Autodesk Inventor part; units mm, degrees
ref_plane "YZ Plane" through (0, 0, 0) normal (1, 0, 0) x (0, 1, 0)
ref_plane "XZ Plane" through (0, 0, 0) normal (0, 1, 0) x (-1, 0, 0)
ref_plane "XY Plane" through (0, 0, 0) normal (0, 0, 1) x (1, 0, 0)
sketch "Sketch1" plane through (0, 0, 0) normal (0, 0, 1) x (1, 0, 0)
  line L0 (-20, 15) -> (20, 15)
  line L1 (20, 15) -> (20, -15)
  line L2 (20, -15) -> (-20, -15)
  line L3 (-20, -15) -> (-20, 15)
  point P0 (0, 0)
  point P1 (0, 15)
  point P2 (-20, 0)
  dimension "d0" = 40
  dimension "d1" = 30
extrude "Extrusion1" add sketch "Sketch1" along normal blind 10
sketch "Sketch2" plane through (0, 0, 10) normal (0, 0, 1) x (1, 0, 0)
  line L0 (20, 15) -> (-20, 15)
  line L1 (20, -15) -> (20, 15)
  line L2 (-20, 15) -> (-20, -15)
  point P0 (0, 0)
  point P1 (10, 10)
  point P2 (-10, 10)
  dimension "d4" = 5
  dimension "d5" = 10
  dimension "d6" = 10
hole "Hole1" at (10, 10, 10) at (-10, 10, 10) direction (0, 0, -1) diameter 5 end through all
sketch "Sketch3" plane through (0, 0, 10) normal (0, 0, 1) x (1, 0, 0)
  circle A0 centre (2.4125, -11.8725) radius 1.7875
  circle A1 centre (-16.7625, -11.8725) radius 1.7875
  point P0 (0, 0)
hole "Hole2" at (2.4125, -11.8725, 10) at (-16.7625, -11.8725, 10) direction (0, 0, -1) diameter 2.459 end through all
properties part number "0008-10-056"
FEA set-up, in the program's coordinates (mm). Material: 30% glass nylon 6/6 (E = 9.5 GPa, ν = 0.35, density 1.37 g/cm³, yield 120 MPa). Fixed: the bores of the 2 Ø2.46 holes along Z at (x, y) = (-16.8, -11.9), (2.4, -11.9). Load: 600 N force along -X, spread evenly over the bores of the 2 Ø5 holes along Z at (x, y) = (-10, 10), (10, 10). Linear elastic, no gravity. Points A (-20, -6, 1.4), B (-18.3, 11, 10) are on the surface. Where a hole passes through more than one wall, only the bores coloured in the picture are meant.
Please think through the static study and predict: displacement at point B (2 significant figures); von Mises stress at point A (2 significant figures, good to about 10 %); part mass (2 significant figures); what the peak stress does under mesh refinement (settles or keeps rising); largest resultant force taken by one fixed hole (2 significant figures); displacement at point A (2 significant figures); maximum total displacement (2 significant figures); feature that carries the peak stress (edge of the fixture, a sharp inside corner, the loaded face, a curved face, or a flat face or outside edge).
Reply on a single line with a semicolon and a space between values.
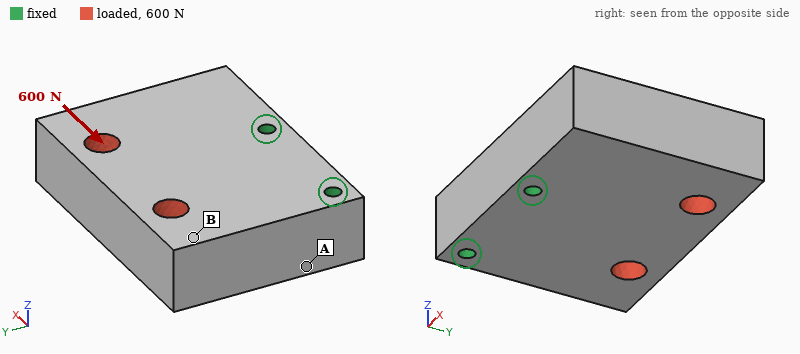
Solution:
34 µm; 6.8 MPa; 16 g; keeps rising; 720 N; 11 µm; 51 µm; edge of the fixture
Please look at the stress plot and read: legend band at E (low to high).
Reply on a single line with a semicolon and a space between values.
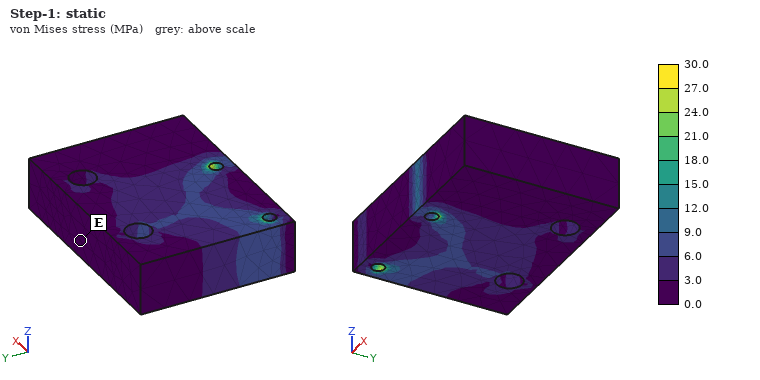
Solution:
0.0 to 3.0 MPa
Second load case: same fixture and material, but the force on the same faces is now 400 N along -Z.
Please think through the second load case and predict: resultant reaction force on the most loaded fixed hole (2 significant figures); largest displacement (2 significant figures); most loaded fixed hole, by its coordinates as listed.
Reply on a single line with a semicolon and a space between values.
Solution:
300 N; 0.14 mm; (2.4, -11.9)
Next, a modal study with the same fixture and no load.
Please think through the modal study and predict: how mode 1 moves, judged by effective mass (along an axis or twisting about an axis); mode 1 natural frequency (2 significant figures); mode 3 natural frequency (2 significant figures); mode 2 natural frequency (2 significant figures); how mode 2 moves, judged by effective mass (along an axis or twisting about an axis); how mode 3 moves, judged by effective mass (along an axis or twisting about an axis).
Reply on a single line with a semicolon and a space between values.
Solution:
along Z; 3900 Hz; 6900 Hz; 6600 Hz; twisting about Y; along X
